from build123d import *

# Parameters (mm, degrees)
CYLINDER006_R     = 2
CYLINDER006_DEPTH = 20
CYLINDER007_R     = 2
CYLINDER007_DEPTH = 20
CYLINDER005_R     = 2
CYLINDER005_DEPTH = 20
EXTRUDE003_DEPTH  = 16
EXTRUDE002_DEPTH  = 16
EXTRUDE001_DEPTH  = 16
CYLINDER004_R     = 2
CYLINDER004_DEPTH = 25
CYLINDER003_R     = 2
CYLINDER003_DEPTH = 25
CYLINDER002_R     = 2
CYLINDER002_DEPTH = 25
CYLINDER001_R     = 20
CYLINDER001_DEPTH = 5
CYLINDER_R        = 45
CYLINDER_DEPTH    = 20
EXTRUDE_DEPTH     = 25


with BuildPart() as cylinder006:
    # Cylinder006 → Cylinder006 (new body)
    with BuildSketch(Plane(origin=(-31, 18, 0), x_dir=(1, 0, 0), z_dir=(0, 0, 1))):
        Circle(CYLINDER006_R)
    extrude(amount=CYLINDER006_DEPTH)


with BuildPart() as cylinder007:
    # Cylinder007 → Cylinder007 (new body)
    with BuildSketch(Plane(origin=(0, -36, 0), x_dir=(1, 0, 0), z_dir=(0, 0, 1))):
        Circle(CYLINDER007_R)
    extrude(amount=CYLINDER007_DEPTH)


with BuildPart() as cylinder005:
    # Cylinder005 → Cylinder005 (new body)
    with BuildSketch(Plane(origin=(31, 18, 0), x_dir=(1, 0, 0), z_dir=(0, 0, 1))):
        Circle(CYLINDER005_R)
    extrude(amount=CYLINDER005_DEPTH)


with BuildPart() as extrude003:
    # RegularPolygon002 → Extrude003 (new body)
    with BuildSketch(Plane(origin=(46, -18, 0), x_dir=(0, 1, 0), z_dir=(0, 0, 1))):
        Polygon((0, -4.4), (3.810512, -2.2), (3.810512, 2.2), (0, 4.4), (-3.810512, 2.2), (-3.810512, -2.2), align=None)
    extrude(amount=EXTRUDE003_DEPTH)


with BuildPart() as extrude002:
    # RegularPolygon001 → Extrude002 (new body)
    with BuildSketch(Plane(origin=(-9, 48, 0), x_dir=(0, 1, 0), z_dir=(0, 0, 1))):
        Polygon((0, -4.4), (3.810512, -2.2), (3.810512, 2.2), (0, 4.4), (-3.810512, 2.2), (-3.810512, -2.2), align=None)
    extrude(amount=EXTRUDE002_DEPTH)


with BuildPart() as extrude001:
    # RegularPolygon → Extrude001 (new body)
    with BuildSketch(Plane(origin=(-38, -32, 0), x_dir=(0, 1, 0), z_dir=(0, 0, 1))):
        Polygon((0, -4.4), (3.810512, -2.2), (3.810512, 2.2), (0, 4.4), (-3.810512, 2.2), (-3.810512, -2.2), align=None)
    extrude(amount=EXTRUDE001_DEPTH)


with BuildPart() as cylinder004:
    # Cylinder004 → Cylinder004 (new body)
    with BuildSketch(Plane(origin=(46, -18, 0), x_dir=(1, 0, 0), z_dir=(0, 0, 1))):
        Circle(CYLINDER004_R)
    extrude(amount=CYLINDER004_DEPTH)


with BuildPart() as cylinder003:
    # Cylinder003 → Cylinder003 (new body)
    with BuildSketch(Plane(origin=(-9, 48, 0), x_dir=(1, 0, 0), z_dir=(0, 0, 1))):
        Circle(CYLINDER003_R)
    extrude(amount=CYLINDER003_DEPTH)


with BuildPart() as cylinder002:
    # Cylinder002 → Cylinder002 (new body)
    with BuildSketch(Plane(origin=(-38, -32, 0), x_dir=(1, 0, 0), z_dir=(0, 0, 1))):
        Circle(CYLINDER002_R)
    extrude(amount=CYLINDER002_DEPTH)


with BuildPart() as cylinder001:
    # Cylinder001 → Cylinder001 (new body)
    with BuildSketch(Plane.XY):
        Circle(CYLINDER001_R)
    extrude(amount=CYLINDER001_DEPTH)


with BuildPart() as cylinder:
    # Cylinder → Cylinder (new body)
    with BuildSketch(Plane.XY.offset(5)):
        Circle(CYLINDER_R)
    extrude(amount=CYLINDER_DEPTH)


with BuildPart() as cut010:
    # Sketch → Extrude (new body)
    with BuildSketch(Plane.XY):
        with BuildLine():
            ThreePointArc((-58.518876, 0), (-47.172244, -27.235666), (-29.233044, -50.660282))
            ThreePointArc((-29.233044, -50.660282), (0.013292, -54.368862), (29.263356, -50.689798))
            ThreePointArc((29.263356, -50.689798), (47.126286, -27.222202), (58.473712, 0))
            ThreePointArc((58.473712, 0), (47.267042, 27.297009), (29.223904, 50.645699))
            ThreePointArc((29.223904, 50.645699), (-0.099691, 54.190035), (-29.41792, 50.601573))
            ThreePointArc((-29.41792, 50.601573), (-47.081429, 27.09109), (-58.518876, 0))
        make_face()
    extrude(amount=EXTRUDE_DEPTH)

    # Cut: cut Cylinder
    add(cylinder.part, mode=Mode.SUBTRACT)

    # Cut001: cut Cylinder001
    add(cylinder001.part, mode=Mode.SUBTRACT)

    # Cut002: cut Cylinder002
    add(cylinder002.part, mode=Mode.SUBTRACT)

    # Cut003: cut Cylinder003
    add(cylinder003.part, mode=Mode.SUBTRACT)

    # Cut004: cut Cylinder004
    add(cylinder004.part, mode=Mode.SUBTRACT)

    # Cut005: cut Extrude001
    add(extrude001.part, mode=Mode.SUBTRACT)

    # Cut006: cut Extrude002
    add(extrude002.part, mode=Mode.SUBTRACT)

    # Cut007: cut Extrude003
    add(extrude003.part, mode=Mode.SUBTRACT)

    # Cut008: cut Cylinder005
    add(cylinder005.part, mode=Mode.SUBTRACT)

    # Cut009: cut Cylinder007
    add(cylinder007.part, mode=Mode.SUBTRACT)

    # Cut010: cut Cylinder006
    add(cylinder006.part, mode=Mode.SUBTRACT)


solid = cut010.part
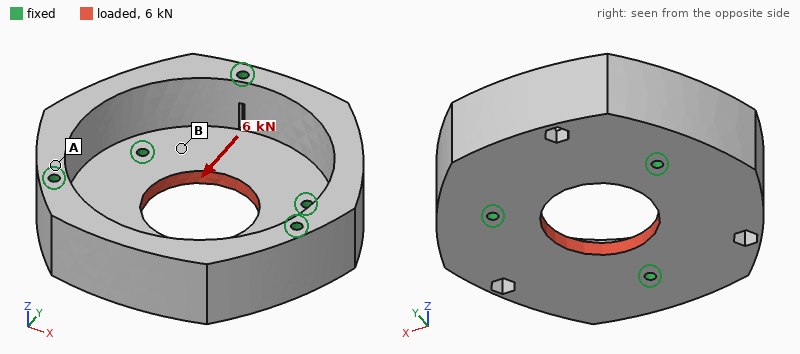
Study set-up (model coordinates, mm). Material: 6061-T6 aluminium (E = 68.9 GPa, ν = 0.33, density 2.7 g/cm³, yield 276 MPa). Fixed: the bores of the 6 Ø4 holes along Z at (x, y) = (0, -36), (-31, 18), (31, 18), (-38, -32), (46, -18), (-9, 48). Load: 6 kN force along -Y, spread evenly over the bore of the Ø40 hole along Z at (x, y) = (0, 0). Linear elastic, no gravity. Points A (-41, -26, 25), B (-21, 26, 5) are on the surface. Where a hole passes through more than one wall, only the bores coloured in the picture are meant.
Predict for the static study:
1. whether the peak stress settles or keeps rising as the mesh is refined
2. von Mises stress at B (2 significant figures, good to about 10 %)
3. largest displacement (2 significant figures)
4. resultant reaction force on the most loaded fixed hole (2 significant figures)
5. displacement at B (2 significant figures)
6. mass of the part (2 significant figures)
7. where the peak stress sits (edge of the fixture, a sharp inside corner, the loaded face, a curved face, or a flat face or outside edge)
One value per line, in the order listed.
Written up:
keeps rising
11 MPa
9.2 µm
1.8 kN
4.4 µm
290 g
edge of the fixture
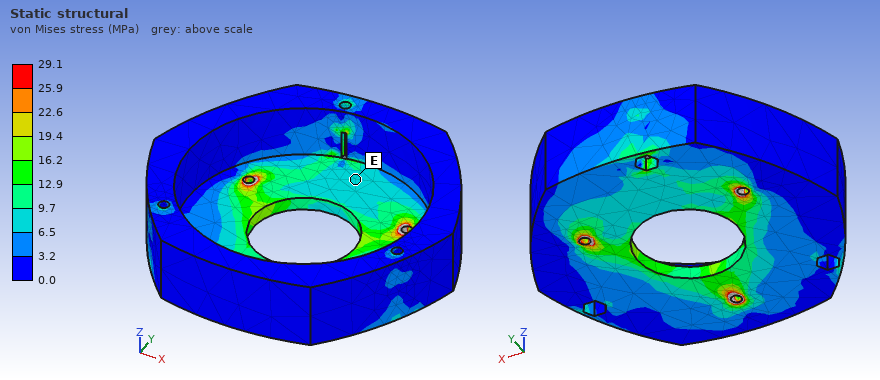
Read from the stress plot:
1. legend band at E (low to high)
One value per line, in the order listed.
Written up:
6.5 to 9.7 MPa
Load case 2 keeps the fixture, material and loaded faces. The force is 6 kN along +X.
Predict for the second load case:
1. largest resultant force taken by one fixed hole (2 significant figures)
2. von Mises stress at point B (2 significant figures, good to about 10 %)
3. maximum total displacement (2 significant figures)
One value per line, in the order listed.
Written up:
1.8 kN
7.5 MPa
8.3 µm
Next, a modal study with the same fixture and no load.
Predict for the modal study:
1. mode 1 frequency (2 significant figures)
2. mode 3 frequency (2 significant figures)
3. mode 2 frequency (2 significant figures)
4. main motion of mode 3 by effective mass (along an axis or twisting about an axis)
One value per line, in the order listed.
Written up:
8200 Hz
8900 Hz
8400 Hz
along Z
